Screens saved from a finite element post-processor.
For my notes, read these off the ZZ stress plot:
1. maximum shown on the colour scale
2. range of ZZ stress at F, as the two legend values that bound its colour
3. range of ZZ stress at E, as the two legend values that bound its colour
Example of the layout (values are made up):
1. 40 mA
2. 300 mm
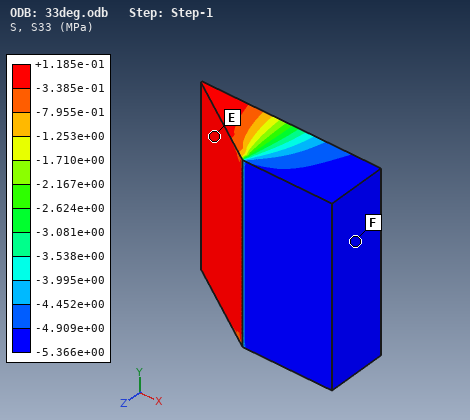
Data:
1. +1.185e-01 MPa
2. -5.366e+00 to -4.909e+00 MPa
3. -3.385e-01 to +1.185e-01 MPa
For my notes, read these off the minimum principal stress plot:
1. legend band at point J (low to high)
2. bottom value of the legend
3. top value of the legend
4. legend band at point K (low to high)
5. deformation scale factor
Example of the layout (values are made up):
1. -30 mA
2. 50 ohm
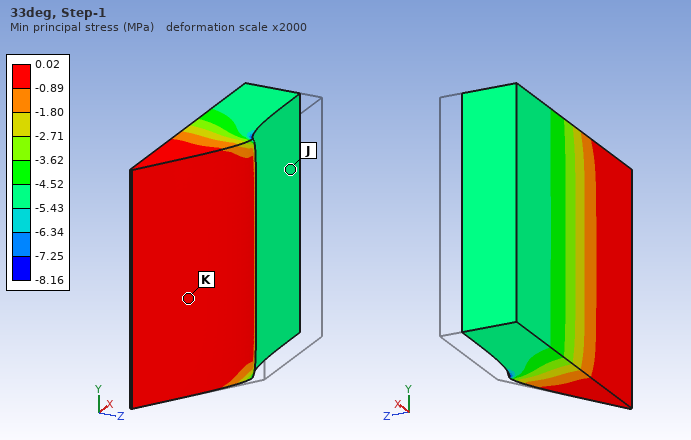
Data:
1. -5.43 to -4.52 MPa
2. -8.16 MPa
3. 0.02 MPa
4. -0.89 to 0.02 MPa
5. 2000
